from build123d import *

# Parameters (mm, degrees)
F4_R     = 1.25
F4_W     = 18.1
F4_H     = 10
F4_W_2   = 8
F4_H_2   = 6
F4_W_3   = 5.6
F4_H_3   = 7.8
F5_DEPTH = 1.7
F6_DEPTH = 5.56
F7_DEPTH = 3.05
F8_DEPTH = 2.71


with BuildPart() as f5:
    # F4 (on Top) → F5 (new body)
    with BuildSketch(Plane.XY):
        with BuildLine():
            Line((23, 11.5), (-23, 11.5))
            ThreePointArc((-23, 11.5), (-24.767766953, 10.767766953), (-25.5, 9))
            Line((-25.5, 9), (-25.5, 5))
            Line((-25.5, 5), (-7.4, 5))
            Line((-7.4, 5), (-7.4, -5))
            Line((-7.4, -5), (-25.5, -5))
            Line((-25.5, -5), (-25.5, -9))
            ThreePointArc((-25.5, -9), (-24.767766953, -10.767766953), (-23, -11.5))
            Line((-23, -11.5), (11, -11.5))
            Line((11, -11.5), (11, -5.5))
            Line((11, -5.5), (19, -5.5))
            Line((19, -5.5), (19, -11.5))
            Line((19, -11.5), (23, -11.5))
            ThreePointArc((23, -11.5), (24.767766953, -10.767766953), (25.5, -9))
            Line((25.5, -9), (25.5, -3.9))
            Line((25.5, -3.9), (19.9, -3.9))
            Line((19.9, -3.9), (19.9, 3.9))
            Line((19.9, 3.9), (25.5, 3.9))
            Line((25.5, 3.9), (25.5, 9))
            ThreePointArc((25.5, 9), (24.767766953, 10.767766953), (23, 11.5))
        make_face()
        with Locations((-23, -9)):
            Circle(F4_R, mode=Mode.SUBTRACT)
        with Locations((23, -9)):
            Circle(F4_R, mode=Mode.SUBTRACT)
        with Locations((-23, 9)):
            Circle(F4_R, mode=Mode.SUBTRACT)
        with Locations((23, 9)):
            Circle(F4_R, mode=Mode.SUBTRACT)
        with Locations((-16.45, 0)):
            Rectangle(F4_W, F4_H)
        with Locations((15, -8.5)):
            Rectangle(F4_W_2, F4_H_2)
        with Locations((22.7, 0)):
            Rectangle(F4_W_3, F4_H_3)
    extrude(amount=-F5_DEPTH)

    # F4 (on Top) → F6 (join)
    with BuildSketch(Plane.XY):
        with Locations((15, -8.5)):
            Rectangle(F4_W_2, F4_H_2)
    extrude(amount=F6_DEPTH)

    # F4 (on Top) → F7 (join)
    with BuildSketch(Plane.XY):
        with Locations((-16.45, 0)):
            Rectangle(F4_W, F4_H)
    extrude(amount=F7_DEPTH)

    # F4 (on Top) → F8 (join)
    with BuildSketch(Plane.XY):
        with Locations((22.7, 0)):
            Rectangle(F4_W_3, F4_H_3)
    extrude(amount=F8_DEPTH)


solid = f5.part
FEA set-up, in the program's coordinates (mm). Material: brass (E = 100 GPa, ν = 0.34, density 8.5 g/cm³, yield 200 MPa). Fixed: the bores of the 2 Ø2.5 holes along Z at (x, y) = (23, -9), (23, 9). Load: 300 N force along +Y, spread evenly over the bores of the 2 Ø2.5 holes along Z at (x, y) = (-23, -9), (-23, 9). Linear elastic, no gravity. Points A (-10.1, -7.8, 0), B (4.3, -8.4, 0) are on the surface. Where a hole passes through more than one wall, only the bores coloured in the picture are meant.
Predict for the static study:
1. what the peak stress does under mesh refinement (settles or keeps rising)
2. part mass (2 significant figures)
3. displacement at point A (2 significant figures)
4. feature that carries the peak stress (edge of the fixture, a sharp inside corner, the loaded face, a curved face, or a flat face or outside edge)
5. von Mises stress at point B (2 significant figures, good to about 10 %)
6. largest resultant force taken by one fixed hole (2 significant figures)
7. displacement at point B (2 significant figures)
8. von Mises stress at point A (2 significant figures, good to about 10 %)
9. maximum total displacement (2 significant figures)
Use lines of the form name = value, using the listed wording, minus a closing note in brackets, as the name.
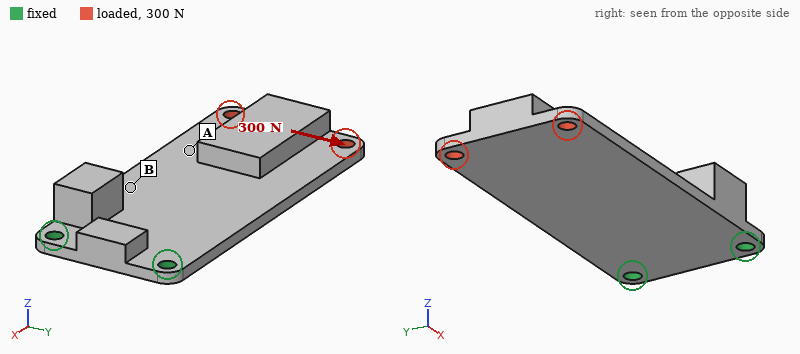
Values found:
what the peak stress does under mesh refinement = keeps rising
part mass = 25 g
displacement at point A = 44 µm
feature that carries the peak stress = edge of the fixture
von Mises stress at point B = 43 MPa
largest resultant force taken by one fixed hole = 760 N
displacement at point B = 20 µm
von Mises stress at point A = 19 MPa
maximum total displacement = 79 µm
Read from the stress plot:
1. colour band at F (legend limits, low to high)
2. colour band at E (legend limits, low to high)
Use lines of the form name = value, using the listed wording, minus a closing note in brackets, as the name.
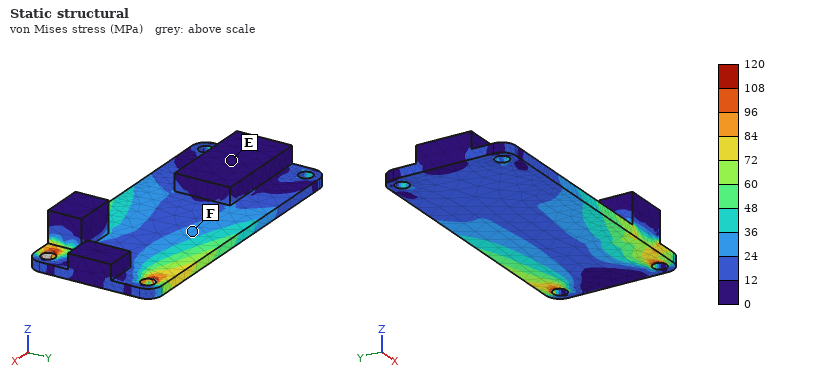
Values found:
colour band at F = 24 to 36 MPa
colour band at E = 0 to 12 MPa
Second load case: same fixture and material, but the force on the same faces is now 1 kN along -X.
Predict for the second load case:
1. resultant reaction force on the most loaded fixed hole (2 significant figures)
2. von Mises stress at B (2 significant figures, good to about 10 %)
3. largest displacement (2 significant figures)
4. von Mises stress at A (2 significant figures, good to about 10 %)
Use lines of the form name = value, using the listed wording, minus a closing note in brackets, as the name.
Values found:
resultant reaction force on the most loaded fixed hole = 510 N
von Mises stress at B = 26 MPa
largest displacement = 29 µm
von Mises stress at A = 22 MPa
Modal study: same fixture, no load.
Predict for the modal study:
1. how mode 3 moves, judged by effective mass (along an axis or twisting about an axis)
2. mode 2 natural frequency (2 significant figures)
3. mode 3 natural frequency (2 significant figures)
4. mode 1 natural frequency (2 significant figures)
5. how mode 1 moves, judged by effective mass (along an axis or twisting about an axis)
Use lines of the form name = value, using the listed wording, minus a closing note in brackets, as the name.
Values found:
how mode 3 moves, judged by effective mass = along Z
mode 2 natural frequency = 2000 Hz
mode 3 natural frequency = 2400 Hz
mode 1 natural frequency = 340 Hz
how mode 1 moves, judged by effective mass = along Z
